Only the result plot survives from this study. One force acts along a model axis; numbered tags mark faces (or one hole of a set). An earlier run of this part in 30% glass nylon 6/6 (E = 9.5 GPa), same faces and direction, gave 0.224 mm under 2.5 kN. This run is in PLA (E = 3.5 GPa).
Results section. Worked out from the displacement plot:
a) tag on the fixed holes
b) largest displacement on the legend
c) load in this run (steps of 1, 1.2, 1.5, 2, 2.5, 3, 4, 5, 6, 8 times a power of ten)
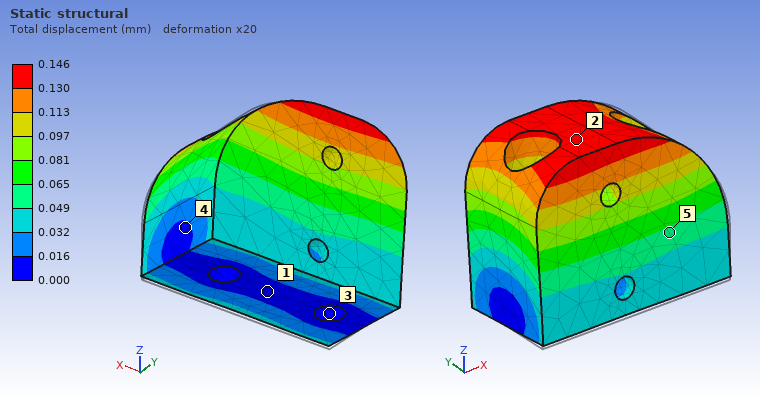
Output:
3
0.146 mm
600 N
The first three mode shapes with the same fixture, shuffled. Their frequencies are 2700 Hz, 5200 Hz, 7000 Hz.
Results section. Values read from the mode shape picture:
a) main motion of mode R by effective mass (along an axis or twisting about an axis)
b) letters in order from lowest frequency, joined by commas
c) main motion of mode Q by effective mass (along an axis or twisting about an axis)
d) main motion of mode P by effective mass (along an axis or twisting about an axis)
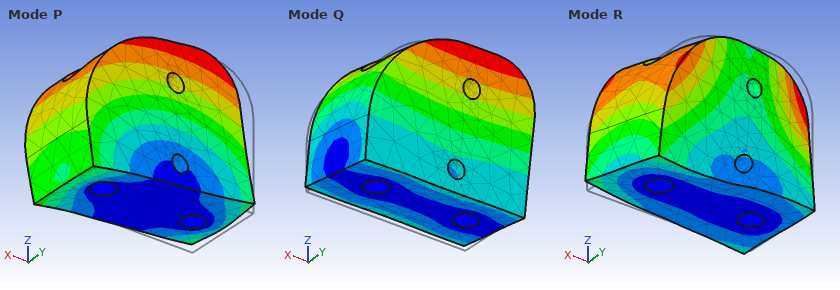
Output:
twisting about Z
Q, P, R
along Y
along X
